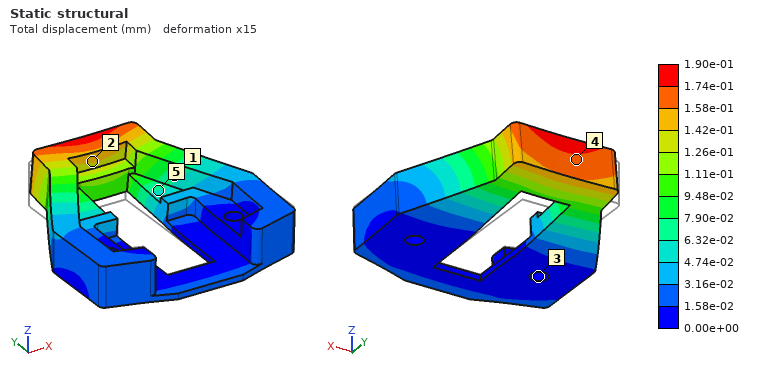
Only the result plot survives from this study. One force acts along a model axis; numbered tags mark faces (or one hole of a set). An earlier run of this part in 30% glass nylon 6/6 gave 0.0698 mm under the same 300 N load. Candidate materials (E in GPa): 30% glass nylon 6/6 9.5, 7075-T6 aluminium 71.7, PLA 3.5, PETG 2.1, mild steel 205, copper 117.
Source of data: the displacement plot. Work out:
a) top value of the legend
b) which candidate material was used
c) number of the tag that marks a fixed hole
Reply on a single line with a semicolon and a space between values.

1.90e-01 mm; PLA; 3
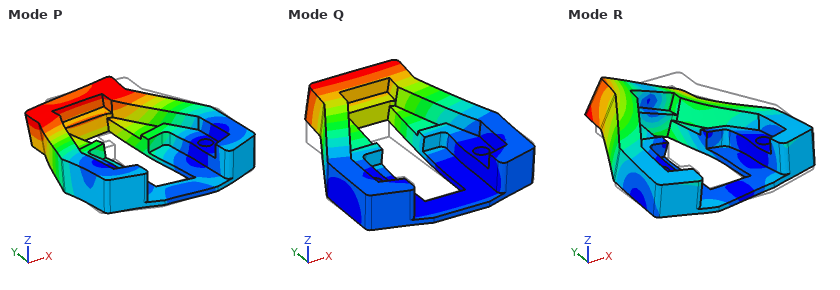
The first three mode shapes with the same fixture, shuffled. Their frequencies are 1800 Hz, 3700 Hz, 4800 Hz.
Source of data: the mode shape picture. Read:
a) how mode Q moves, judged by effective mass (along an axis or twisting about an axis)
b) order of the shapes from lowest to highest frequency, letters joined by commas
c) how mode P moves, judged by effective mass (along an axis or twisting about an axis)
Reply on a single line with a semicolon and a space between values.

along Z; Q, P, R; along X
